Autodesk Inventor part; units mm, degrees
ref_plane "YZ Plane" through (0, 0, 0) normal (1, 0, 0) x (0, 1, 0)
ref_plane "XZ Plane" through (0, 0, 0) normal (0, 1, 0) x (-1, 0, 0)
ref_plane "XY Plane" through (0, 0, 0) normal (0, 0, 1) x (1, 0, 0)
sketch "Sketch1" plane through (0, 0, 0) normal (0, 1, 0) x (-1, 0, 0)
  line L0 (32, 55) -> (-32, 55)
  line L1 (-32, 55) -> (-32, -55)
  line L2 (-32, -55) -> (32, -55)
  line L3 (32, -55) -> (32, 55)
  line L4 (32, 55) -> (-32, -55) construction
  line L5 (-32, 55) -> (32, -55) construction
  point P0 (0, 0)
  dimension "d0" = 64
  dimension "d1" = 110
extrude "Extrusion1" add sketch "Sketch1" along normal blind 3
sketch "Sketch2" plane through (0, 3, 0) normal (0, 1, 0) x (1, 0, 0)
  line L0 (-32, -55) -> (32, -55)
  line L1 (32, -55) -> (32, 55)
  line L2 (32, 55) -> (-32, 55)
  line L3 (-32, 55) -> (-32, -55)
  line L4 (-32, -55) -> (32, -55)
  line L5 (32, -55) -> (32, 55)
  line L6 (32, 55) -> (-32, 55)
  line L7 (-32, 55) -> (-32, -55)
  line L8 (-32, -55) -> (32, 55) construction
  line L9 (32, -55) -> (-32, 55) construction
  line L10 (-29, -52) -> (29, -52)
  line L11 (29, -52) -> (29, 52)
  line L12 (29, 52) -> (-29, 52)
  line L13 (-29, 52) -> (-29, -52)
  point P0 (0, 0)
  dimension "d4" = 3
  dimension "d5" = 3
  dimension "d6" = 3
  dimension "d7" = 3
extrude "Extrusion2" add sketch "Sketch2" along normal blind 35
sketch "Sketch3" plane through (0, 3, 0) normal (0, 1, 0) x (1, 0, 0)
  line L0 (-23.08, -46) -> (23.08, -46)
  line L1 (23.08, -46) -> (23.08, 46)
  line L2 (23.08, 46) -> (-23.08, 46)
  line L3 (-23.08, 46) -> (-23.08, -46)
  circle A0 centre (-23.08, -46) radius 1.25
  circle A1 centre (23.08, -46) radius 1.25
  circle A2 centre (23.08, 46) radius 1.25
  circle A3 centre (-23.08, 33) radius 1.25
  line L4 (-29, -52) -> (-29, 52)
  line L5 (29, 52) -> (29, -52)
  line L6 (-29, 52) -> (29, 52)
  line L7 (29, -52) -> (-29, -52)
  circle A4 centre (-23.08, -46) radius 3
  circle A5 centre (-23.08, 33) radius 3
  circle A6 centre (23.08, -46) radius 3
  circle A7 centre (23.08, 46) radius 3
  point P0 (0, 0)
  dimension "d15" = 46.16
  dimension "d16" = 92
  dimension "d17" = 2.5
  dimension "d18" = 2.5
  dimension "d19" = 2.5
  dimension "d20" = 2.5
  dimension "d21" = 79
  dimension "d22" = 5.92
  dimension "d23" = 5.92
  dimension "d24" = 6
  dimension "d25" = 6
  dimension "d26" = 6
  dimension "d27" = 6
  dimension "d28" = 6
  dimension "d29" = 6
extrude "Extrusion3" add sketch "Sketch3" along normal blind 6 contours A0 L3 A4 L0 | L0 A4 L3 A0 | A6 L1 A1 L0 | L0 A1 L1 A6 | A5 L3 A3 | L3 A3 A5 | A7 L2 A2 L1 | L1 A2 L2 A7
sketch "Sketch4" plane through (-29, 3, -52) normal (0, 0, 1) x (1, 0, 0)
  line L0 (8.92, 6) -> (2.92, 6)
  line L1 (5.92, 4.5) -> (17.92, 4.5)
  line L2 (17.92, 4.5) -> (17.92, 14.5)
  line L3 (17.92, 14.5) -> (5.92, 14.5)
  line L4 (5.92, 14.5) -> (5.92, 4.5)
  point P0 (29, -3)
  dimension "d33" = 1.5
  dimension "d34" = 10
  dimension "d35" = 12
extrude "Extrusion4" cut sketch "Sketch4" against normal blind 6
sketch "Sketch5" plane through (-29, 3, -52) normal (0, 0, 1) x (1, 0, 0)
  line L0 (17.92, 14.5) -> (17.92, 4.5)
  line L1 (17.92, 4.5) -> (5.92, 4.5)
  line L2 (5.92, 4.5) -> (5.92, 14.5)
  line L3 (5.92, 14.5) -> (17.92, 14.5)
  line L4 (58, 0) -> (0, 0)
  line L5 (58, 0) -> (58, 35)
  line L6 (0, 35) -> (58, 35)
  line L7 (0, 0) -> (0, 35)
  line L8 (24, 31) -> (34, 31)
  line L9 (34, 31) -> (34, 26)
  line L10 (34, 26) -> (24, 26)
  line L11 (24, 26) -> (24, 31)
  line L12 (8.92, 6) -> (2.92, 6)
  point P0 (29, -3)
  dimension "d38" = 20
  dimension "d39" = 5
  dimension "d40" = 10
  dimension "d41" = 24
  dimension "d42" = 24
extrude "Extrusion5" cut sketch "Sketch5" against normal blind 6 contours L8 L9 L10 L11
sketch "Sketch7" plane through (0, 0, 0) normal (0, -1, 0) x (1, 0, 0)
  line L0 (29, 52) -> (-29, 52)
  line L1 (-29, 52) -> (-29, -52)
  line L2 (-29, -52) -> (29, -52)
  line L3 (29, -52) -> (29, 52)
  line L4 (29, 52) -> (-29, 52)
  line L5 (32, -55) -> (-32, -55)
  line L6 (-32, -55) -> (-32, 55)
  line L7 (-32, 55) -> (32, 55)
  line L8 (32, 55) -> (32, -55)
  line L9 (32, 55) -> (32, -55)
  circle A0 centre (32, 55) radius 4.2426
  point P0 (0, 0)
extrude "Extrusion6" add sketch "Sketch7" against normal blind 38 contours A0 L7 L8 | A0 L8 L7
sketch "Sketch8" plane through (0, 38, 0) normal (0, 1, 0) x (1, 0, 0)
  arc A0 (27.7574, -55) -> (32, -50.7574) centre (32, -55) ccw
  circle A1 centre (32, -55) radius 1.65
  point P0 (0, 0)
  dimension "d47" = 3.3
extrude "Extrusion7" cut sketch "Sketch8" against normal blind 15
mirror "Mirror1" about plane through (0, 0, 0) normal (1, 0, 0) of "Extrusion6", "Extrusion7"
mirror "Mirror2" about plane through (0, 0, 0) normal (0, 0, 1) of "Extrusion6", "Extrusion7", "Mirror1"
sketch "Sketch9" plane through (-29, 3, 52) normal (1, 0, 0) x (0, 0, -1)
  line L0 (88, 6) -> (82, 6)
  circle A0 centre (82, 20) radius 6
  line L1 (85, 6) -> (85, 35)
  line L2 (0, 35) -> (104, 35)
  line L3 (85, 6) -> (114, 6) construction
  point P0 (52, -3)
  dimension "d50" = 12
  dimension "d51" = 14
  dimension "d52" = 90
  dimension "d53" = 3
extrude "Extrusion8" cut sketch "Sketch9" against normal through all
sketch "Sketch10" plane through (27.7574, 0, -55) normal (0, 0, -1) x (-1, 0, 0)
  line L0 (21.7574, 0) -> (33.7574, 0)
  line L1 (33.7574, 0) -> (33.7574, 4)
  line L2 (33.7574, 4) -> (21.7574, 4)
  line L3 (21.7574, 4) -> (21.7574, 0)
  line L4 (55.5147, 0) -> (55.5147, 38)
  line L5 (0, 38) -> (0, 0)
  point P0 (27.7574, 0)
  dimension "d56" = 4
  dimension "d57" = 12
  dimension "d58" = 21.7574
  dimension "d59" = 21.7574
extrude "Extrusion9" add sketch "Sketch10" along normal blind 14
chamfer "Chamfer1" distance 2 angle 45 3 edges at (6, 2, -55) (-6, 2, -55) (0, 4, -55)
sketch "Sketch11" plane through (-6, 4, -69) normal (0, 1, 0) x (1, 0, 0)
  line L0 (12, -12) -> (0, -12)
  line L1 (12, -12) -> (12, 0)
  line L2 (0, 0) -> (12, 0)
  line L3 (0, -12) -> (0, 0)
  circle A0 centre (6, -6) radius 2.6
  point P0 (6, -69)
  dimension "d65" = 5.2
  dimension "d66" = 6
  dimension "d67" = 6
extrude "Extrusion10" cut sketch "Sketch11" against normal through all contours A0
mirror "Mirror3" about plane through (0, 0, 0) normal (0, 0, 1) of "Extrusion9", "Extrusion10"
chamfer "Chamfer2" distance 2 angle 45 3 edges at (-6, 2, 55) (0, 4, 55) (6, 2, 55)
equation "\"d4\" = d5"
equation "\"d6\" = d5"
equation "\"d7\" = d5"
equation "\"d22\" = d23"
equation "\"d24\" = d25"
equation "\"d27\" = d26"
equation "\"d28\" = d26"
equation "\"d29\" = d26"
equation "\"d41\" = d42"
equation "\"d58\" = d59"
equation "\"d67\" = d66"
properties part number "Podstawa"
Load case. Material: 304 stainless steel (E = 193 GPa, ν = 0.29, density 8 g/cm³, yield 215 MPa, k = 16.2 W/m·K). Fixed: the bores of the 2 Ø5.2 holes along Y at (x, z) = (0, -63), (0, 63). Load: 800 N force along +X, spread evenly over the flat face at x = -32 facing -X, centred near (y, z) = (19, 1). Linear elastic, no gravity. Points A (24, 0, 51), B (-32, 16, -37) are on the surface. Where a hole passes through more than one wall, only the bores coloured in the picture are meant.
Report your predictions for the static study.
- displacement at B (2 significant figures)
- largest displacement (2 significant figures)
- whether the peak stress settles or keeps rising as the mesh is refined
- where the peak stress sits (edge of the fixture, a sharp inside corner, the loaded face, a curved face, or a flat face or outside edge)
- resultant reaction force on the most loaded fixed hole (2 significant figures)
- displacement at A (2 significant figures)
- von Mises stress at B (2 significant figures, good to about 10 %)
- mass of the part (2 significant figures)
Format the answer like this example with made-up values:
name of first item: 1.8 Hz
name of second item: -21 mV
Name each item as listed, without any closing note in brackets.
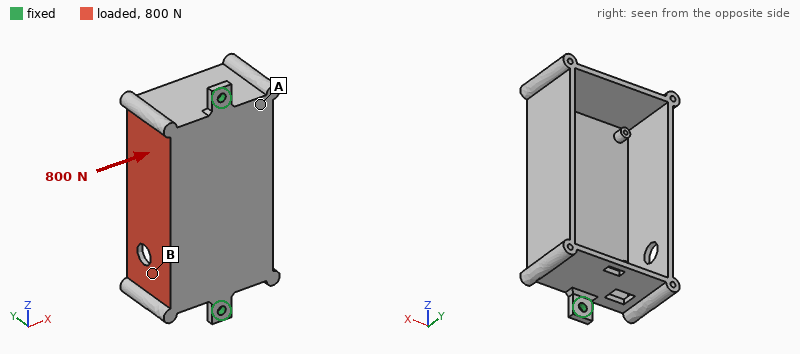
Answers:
displacement at B: 0.080 mm
largest displacement: 0.18 mm
whether the peak stress settles or keeps rising as the mesh is refined: keeps rising
where the peak stress sits: edge of the fixture
resultant reaction force on the most loaded fixed hole: 410 N
displacement at A: 0.051 mm
von Mises stress at B: 25 MPa
mass of the part: 510 g
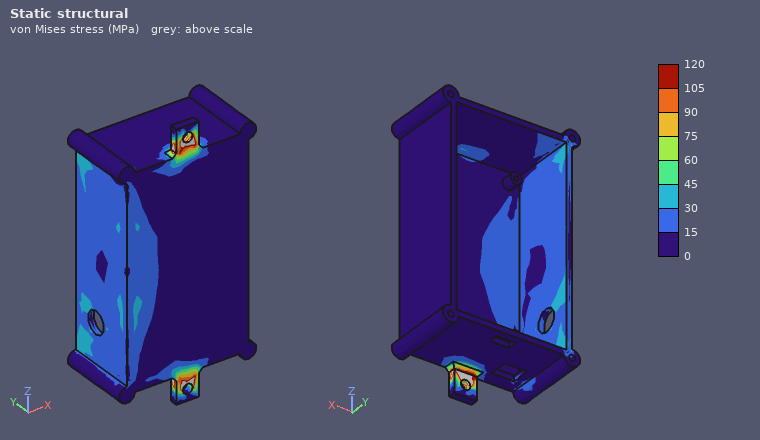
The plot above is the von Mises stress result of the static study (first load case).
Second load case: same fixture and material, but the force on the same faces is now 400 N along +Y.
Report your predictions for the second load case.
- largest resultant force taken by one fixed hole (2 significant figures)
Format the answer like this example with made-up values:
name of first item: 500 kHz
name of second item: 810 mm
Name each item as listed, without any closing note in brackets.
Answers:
largest resultant force taken by one fixed hole: 200 N
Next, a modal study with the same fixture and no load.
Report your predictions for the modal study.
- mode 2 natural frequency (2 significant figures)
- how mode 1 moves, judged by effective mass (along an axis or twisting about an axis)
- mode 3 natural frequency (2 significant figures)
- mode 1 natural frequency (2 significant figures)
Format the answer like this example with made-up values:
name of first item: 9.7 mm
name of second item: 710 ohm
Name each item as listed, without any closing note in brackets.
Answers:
mode 2 natural frequency: 1100 Hz
how mode 1 moves, judged by effective mass: along X
mode 3 natural frequency: 2000 Hz
mode 1 natural frequency: 600 Hz
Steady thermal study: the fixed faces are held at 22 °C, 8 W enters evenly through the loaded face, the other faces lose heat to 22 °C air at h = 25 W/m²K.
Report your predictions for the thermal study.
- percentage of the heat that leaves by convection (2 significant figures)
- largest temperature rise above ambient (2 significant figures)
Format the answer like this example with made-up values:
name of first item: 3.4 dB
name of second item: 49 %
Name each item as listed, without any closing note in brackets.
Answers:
percentage of the heat that leaves by convection: 91 %
largest temperature rise above ambient: 32 K
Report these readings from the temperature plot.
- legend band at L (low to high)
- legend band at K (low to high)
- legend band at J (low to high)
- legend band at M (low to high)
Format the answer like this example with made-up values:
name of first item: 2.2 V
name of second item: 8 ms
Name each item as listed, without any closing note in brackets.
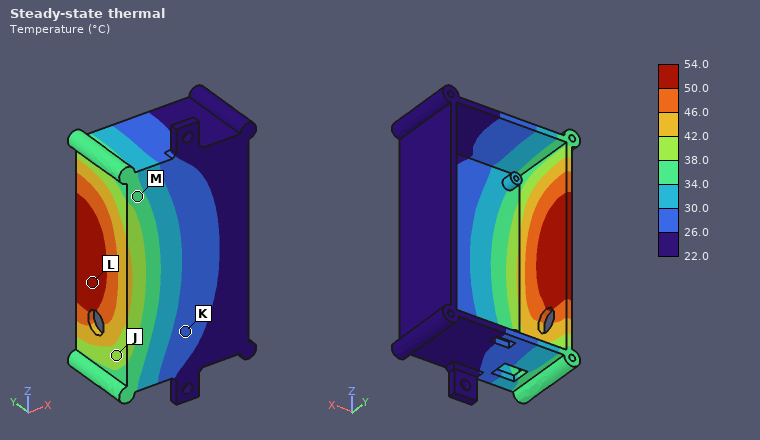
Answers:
legend band at L: 50.0 to 54.0 °C
legend band at K: 26.0 to 30.0 °C
legend band at J: 38.0 to 42.0 °C
legend band at M: 34.0 to 38.0 °C
